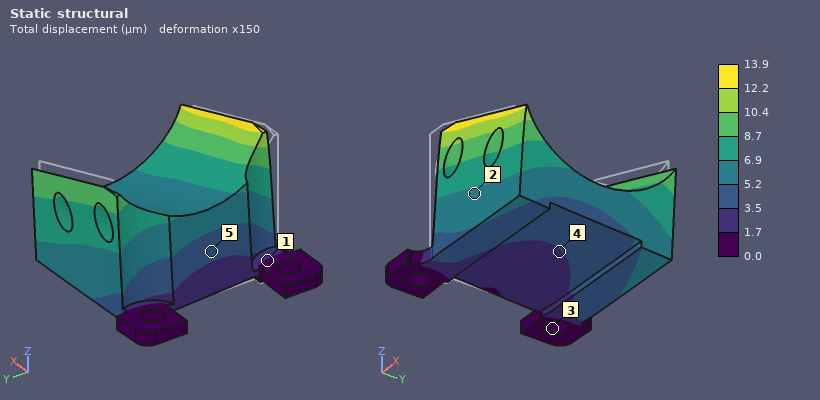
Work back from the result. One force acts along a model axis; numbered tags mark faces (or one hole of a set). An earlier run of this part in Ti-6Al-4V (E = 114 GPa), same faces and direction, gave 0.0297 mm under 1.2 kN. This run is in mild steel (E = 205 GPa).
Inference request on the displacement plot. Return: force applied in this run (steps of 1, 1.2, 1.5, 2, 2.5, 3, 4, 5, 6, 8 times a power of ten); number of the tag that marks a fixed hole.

1 kN
3
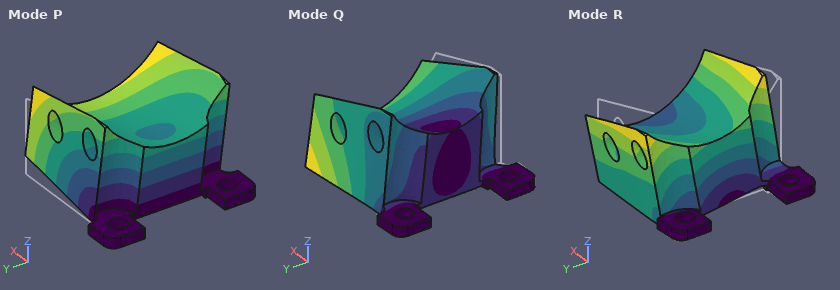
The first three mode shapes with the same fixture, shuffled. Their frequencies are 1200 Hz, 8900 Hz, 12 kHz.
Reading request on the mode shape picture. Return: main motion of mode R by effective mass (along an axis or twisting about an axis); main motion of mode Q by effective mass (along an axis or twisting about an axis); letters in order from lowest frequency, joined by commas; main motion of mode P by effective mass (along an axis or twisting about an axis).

along Y
along Y
P, R, Q
along Z
